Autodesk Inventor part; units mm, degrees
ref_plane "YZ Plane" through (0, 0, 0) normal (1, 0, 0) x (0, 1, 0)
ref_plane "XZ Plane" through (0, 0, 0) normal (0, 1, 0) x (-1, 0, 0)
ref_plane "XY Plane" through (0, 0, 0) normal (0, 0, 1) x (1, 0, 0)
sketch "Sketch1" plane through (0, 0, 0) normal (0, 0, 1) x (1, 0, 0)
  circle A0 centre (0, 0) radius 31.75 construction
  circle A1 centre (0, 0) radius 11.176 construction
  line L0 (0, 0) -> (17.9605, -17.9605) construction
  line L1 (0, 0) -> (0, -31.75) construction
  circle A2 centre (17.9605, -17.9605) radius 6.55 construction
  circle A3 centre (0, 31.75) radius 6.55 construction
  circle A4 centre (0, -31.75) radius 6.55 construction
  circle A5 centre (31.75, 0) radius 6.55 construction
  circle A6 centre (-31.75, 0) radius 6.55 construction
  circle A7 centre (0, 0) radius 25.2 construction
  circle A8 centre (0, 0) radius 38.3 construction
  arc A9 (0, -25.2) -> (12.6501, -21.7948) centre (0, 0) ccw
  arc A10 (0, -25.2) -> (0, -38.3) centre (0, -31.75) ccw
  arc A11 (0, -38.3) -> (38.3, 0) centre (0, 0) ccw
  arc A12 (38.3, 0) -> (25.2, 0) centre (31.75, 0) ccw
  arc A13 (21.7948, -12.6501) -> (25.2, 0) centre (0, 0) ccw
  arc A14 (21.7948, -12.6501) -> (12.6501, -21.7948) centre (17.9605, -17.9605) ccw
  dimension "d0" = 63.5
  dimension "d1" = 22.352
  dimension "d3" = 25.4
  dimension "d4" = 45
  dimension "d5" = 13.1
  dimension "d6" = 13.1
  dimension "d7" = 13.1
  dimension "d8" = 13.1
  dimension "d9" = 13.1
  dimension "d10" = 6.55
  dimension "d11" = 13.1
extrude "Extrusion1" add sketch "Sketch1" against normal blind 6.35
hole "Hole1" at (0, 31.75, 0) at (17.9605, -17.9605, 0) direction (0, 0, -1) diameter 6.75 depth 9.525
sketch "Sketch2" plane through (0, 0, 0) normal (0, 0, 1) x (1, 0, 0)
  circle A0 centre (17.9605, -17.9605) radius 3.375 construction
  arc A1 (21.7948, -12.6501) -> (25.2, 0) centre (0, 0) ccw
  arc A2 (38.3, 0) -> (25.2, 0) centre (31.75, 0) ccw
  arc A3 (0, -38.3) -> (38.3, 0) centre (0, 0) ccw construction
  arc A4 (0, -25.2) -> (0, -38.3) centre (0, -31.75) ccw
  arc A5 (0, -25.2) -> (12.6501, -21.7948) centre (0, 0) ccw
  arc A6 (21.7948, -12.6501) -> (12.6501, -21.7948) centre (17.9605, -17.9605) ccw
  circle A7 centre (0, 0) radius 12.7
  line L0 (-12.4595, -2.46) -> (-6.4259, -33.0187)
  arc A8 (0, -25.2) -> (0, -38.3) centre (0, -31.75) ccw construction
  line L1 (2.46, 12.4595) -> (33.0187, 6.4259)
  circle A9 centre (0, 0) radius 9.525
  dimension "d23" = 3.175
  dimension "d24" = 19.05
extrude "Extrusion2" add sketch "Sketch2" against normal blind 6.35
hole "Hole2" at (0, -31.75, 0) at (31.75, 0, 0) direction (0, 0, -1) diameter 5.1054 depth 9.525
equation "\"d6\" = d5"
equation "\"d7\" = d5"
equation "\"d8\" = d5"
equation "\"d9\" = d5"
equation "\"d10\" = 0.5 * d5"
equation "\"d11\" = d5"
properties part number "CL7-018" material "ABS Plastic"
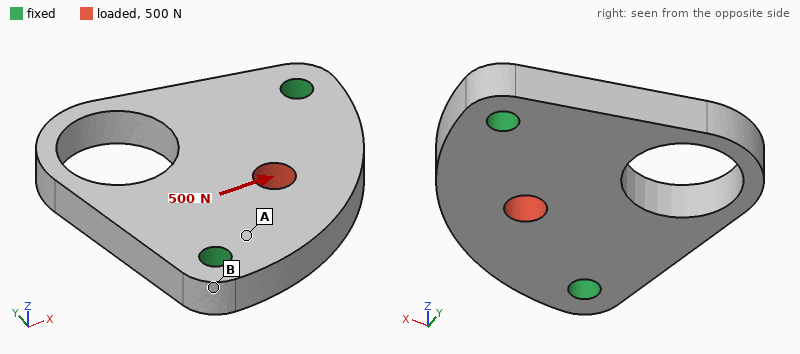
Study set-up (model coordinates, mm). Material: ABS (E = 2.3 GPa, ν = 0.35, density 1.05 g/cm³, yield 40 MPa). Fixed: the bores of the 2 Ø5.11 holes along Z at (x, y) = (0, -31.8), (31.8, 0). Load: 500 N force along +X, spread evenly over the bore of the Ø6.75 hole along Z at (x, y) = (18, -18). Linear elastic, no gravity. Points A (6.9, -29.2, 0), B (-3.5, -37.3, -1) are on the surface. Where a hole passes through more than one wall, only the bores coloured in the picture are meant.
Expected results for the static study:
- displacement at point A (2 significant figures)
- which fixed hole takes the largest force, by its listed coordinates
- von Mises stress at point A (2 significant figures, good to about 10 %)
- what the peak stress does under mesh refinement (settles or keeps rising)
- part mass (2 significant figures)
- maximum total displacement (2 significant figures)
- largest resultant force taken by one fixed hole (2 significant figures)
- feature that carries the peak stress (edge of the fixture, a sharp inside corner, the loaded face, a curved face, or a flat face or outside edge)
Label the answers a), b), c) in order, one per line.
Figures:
a) 14 µm
b) (0, -31.8)
c) 4.0 MPa
d) keeps rising
e) 11 g
f) 51 µm
g) 270 N
h) edge of the fixture
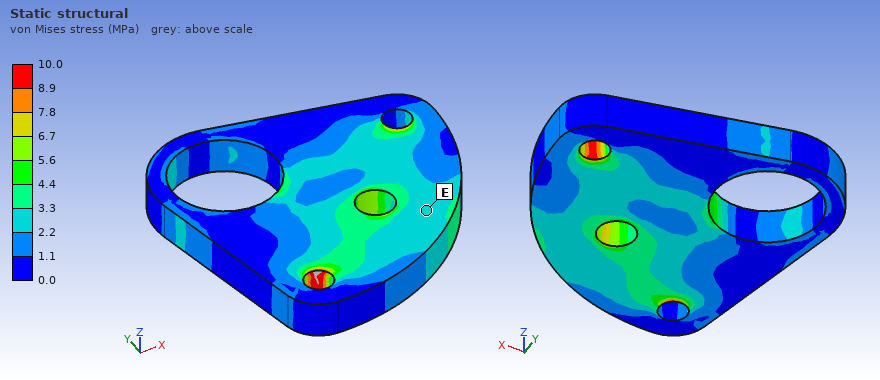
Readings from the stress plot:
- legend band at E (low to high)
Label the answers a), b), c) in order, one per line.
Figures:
a) 2.2 to 3.3 MPa
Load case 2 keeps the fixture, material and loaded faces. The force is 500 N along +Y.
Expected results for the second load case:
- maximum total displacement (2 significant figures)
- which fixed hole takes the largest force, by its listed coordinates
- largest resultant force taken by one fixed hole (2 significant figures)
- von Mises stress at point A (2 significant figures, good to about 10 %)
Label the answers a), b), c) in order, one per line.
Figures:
a) 51 µm
b) (31.8, 0)
c) 270 N
d) 2.6 MPa
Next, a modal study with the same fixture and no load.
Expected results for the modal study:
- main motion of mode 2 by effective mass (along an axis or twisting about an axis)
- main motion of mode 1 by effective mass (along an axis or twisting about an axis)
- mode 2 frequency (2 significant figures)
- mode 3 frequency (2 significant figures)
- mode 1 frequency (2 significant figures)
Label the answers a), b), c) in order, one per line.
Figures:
a) along Z
b) along Z
c) 3600 Hz
d) 4000 Hz
e) 1700 Hz
